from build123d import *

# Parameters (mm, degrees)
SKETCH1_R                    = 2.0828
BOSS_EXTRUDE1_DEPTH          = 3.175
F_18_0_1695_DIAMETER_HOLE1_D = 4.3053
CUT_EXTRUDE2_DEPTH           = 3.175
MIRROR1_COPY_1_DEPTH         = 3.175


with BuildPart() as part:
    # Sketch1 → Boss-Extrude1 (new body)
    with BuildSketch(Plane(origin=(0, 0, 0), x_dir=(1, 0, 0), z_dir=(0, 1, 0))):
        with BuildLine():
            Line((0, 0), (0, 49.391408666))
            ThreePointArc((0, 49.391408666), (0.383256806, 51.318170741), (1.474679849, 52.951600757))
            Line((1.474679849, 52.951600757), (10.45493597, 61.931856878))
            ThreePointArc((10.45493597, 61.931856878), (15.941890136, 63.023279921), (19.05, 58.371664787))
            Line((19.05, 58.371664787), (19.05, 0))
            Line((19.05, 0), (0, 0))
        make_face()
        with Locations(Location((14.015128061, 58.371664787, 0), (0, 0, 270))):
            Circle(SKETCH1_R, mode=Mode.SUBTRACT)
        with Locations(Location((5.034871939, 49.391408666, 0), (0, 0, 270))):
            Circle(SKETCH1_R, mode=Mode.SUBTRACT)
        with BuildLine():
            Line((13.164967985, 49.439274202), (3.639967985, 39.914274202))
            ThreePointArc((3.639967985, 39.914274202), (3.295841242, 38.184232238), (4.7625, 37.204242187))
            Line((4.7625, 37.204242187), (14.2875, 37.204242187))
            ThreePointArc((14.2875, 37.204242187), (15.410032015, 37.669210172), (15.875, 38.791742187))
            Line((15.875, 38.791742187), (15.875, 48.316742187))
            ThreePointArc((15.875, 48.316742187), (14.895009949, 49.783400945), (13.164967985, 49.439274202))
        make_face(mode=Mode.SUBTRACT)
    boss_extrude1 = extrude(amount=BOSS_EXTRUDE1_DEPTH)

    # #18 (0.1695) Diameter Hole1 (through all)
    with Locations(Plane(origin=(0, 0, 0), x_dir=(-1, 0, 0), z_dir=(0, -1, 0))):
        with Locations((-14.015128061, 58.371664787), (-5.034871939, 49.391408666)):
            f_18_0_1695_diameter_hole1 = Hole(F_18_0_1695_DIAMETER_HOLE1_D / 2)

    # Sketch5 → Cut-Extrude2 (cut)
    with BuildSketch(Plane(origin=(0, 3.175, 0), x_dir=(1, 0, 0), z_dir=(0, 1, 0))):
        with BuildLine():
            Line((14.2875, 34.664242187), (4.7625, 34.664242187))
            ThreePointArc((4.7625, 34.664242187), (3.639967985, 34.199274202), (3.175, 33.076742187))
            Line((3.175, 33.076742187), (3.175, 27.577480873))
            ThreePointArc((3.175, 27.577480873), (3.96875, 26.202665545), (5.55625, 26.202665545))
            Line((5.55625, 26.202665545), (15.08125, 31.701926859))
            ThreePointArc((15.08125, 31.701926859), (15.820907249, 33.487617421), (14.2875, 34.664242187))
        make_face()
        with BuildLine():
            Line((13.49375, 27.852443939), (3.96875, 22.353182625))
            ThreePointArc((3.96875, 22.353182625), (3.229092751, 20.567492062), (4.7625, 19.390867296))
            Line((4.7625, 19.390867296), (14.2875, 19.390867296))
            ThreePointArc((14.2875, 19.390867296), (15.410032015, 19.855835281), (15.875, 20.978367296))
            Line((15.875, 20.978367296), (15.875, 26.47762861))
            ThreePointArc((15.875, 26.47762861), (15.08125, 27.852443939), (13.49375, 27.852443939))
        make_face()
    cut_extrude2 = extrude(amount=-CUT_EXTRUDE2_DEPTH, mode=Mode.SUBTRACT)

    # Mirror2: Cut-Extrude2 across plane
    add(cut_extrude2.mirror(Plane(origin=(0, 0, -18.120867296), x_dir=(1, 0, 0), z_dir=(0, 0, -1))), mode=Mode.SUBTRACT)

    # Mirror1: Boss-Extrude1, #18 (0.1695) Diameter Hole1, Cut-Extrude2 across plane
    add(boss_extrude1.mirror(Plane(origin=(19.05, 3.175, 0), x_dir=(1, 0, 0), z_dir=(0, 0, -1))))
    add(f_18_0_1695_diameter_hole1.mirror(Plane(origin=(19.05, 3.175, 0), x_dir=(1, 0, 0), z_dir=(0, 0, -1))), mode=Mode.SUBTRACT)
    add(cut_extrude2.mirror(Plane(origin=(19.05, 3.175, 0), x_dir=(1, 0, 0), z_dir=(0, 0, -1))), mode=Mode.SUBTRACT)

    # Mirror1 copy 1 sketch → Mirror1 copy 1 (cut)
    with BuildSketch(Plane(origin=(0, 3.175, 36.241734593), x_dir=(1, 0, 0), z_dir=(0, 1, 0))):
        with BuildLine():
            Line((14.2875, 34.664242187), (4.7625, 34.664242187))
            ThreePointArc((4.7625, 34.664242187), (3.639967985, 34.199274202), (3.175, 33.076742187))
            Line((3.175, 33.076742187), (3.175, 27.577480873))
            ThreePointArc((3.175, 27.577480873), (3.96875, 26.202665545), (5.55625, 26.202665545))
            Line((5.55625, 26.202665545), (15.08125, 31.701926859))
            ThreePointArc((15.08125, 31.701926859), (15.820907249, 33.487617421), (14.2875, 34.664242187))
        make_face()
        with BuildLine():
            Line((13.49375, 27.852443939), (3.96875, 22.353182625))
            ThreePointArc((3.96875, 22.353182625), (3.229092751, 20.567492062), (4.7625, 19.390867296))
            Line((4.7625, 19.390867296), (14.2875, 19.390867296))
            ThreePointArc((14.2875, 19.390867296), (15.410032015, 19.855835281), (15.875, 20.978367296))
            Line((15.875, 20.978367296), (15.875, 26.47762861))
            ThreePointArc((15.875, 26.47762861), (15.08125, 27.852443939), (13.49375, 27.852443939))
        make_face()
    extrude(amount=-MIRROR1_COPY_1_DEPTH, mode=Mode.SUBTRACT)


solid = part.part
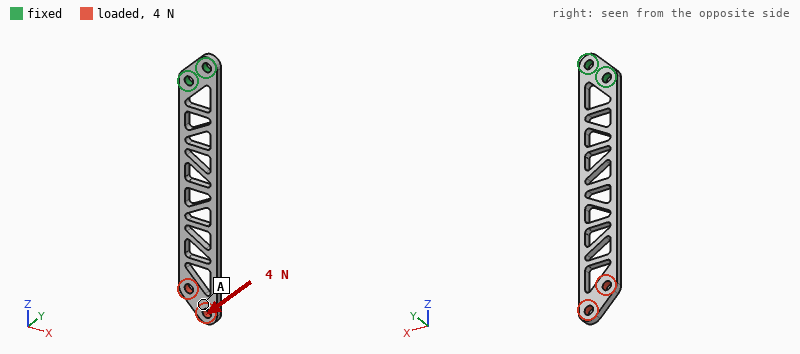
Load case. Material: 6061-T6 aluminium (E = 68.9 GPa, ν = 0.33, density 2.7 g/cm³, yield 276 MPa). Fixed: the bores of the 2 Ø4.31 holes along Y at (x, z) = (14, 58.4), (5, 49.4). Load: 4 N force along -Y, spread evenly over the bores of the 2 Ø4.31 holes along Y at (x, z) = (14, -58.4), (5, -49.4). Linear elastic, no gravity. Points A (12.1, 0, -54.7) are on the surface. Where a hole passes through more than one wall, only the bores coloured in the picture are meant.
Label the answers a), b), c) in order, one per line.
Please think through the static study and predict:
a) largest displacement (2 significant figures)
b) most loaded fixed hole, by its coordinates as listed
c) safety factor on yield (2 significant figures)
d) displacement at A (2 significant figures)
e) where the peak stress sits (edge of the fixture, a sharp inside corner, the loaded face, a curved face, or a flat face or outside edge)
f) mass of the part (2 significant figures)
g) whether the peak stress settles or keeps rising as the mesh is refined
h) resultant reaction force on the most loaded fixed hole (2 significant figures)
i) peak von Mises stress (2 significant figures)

a) 1.2 mm
b) (5, 49.4)
c) 4.4
d) 1.1 mm
e) a curved face
f) 12 g
g) settles
h) 13 N
i) 63 MPa
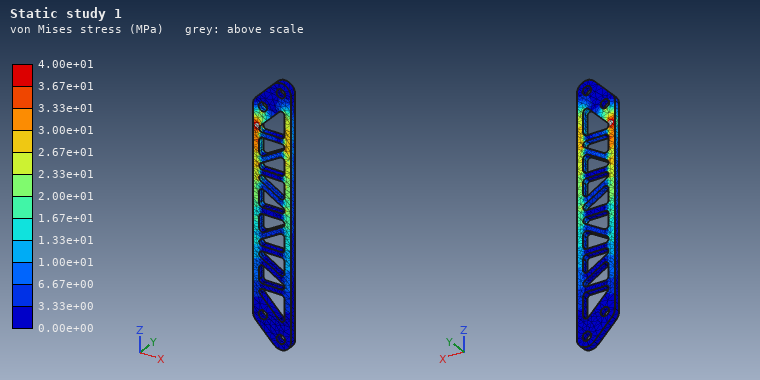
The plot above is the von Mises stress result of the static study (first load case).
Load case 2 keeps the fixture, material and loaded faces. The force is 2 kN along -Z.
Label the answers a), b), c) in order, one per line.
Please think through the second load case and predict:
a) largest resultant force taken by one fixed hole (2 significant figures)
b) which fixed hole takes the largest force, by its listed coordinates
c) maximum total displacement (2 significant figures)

a) 1.1 kN
b) (5, 49.4)
c) 0.17 mm
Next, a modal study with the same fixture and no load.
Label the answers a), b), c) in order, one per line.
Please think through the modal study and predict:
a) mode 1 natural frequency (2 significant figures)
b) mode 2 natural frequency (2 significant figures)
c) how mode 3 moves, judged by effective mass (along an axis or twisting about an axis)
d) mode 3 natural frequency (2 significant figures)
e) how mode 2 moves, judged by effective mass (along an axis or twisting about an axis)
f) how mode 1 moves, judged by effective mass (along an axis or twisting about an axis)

a) 170 Hz
b) 1100 Hz
c) along X
d) 1100 Hz
e) along Y
f) along Y
